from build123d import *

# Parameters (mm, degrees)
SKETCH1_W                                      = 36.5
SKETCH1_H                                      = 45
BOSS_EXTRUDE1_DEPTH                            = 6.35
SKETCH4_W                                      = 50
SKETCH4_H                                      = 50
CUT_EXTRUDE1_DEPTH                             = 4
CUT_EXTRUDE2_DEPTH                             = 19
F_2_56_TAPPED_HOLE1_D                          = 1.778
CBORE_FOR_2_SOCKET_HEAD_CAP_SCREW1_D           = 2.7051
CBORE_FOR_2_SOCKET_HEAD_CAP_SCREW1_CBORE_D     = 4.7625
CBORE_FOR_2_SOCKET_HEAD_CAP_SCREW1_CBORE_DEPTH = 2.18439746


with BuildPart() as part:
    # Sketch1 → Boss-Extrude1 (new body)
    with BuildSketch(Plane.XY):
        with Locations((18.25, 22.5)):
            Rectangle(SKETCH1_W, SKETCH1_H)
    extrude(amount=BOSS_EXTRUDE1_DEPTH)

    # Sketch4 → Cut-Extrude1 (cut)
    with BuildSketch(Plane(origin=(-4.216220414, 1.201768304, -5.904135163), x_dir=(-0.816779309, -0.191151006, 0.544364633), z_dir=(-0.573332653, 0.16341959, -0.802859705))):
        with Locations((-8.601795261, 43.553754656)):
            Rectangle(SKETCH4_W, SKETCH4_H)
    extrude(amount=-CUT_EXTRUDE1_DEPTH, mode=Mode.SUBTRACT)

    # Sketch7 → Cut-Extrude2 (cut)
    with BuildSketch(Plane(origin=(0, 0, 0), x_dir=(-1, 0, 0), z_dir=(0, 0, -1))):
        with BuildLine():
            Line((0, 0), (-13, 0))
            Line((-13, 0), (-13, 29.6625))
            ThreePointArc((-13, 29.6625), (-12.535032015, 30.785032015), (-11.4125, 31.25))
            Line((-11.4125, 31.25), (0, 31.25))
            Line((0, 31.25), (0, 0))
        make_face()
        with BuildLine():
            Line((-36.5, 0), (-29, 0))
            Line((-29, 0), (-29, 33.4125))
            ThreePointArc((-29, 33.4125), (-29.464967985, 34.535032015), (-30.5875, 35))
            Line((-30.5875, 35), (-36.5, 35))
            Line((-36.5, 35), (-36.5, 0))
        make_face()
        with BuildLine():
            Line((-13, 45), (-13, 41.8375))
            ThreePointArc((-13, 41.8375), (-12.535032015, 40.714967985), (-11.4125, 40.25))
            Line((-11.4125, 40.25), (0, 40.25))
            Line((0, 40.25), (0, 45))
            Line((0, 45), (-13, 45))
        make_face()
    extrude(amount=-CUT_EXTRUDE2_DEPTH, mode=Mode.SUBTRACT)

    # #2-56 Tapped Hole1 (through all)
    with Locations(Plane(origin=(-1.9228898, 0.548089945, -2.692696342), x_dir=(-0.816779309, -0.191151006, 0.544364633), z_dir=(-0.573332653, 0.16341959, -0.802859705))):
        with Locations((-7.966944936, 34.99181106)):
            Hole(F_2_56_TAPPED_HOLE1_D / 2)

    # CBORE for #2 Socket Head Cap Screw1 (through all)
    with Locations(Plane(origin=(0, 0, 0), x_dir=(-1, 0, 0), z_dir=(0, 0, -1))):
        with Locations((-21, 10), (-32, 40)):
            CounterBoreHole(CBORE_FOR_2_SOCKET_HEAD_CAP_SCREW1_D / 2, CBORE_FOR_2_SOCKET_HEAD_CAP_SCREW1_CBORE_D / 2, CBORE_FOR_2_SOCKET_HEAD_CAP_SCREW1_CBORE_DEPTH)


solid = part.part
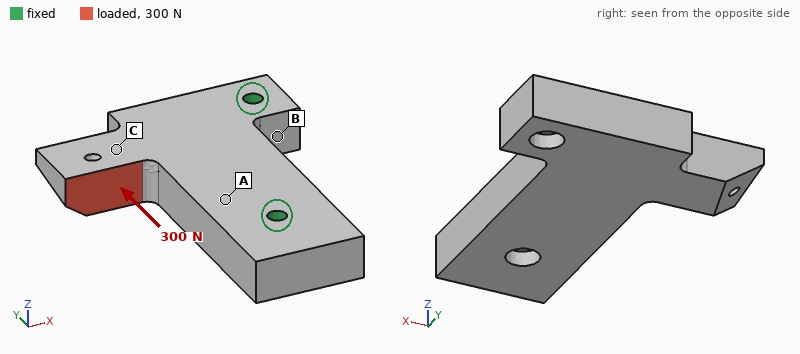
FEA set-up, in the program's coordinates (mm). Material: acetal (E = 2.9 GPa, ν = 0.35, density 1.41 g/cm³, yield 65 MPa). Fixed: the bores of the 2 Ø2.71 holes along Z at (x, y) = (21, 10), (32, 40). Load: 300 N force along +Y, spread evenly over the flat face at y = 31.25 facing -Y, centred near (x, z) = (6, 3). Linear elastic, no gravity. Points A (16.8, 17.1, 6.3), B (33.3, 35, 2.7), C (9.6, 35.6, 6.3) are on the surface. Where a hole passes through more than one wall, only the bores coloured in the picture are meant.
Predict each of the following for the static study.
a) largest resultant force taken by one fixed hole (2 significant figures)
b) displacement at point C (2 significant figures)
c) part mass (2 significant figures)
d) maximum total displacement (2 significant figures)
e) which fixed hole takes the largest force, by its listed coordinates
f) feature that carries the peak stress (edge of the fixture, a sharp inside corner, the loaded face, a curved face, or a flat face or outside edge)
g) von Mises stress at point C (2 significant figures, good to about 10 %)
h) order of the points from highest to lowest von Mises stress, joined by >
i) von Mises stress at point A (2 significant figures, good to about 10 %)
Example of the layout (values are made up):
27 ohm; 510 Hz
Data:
350 N; 0.13 mm; 7.9 g; 0.32 mm; (21, 10); a curved face; 12 MPa; C > A > B; 7.5 MPa
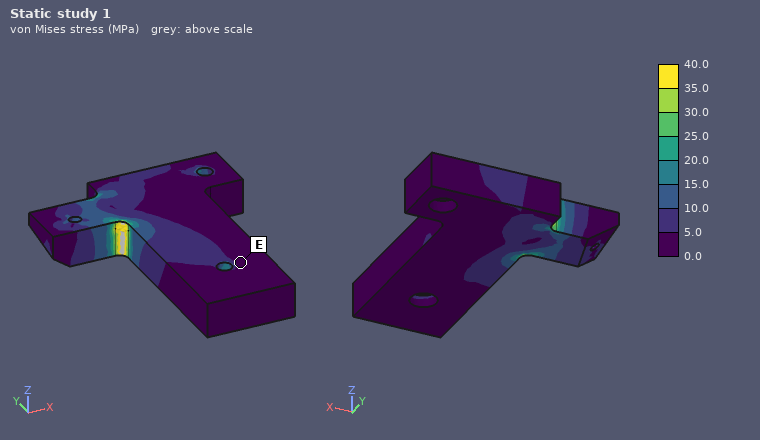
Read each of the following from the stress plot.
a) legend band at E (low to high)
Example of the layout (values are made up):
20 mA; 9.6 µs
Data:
0.0 to 5.0 MPa
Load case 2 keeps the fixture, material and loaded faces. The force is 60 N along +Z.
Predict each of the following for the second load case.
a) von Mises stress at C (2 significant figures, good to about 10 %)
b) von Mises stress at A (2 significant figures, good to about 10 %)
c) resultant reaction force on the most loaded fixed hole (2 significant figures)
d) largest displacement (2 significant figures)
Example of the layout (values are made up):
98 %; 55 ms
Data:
5.7 MPa; 5.0 MPa; 34 N; 0.53 mm
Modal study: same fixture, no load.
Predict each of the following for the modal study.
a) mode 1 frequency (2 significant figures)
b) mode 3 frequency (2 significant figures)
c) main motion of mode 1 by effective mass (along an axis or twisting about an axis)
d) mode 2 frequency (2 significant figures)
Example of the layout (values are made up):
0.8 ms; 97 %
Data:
1700 Hz; 6000 Hz; along Z; 5400 Hz
